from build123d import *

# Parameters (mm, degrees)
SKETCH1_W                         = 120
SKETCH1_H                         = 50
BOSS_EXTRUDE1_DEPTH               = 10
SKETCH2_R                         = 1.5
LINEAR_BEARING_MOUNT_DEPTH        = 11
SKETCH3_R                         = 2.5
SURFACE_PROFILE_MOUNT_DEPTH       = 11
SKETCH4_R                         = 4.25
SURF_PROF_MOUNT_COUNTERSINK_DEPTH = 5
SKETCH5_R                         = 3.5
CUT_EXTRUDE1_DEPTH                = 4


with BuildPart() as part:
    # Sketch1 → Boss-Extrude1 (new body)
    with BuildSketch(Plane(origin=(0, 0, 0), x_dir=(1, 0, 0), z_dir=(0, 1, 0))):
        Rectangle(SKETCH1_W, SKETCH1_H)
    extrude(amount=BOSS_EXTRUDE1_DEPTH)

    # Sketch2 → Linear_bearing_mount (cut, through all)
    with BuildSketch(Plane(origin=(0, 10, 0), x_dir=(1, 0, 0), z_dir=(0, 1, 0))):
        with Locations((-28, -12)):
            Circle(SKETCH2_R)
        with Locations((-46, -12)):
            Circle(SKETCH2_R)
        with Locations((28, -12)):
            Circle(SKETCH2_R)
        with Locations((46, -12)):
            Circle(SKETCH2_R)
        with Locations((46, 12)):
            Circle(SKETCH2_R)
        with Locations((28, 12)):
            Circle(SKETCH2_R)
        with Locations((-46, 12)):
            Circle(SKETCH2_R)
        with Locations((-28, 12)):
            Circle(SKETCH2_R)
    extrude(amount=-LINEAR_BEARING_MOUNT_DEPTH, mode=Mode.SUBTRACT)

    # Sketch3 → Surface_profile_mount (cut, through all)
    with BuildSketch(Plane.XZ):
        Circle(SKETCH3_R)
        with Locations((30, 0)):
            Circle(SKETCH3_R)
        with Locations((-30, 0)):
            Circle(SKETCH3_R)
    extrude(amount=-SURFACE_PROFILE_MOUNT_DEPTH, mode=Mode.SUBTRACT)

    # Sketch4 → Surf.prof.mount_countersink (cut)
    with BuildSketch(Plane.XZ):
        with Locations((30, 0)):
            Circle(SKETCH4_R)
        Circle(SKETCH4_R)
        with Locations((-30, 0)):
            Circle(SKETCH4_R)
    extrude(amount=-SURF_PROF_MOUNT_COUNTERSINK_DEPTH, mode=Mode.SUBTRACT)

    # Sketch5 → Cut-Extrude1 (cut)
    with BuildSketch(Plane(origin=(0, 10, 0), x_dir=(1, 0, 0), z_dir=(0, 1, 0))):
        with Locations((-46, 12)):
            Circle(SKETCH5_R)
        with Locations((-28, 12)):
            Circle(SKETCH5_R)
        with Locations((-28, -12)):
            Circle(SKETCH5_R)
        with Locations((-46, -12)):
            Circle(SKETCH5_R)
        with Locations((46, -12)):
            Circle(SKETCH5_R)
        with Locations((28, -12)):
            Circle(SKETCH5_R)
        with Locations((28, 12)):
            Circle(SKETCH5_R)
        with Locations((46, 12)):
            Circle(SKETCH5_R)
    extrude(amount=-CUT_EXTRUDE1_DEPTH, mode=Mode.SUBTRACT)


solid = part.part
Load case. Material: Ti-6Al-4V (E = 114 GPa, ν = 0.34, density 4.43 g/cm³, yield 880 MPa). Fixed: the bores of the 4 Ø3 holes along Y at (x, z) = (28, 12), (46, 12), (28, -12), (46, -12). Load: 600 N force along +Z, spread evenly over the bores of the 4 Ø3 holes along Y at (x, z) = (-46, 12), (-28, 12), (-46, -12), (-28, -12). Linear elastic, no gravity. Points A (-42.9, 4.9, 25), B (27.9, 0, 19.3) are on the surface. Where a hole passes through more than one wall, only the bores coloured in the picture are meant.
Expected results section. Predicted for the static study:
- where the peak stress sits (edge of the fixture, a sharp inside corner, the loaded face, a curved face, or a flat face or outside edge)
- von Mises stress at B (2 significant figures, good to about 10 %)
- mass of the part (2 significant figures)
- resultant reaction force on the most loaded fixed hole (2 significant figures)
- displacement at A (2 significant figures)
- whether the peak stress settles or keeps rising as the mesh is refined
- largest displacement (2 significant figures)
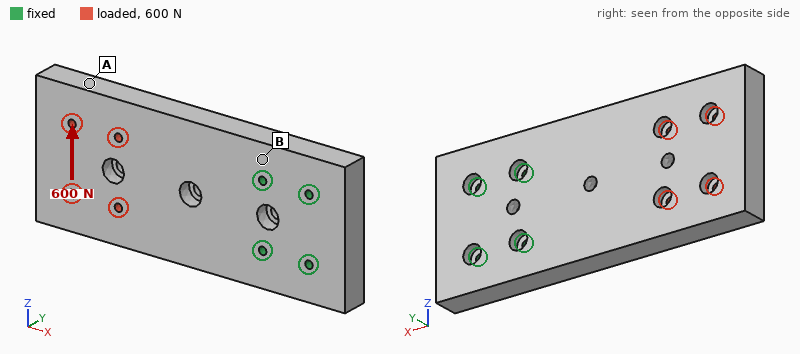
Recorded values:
edge of the fixture
5.3 MPa
250 g
970 N
13 µm
keeps rising
16 µm
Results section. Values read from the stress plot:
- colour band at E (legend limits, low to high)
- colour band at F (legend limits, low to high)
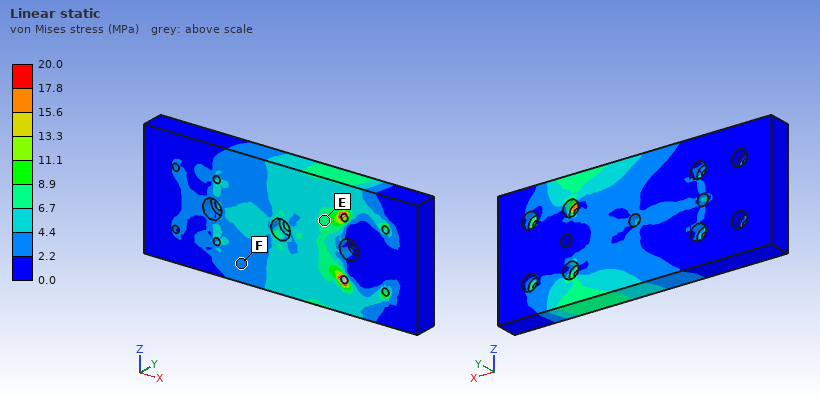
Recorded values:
6.7 to 8.9 MPa
2.2 to 4.4 MPa
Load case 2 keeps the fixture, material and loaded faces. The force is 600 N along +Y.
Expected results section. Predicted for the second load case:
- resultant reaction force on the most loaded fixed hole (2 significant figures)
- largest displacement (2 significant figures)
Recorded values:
1.2 kN
0.24 mm
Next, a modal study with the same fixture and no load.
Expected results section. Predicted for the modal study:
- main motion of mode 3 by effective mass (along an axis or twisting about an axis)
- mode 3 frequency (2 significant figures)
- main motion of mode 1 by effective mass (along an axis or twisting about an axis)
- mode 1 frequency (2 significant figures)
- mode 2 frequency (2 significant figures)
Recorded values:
along Z
3600 Hz
along Y
920 Hz
3300 Hz
